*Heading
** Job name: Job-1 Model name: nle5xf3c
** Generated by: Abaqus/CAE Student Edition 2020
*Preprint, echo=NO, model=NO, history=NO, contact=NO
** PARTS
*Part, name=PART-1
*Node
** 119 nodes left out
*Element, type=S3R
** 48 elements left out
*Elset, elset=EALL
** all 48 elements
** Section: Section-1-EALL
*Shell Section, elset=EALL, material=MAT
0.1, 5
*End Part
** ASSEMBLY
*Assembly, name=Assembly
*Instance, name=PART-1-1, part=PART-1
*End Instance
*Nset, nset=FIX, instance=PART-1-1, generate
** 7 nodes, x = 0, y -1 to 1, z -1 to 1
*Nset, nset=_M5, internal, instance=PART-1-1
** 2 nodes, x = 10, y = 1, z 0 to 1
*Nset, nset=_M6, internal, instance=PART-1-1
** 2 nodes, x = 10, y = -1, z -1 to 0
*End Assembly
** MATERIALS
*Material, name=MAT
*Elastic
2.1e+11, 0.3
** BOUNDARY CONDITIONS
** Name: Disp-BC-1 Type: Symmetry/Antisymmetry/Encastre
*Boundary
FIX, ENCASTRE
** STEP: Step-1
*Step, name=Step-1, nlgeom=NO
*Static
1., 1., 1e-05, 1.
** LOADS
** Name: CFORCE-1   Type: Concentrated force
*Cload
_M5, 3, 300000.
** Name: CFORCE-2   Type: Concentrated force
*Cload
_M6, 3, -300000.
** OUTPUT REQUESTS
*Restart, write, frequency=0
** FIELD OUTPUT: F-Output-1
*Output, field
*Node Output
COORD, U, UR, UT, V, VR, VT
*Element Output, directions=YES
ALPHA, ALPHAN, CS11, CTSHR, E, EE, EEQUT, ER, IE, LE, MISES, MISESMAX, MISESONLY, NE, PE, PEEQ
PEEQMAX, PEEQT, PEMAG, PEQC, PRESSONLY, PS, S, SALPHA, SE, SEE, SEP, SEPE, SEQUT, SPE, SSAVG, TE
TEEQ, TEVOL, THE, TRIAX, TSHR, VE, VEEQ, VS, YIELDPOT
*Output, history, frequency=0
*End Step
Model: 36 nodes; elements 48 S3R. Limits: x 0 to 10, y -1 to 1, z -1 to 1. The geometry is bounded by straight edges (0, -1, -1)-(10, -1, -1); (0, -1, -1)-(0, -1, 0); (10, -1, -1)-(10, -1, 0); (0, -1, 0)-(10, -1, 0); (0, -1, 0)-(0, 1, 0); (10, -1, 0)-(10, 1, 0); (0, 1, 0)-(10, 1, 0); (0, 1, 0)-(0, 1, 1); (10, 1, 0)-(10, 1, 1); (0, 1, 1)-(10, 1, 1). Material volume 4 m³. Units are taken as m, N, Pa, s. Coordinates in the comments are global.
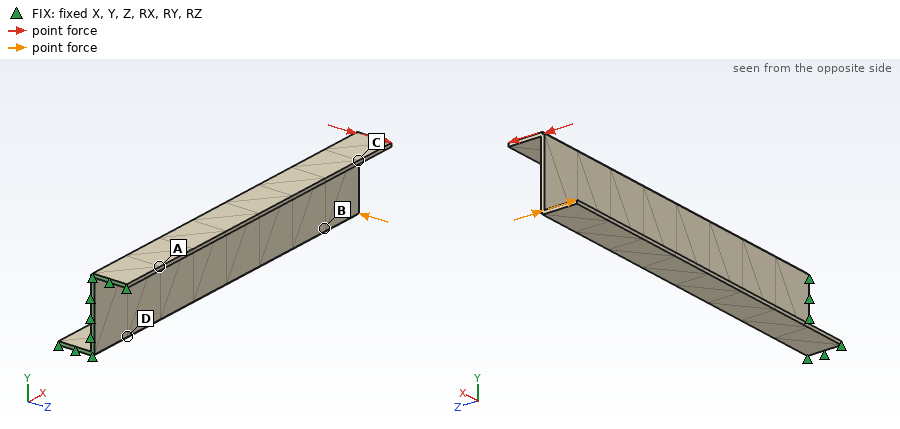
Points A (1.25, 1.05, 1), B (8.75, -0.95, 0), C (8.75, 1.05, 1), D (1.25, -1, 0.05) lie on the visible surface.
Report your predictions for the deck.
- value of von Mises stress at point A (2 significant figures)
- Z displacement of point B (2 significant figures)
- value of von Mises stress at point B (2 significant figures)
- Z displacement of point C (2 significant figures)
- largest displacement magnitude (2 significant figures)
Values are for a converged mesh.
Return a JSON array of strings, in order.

["1.3e+08 Pa", "-0.025 m", "4.3e+07 Pa", "0.027 m", "0.044 m"]
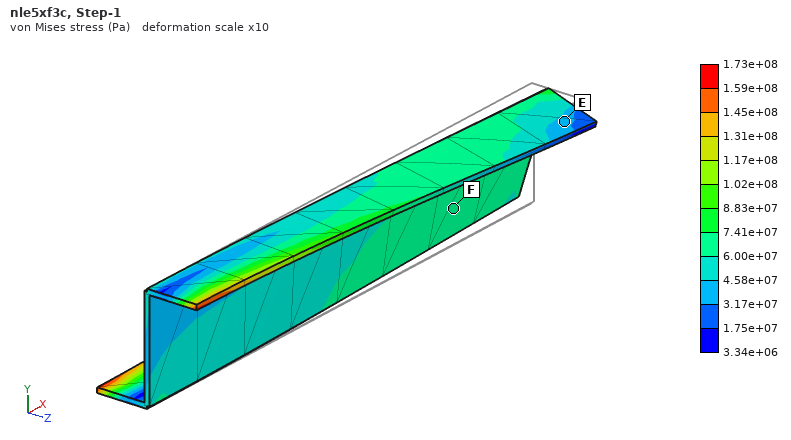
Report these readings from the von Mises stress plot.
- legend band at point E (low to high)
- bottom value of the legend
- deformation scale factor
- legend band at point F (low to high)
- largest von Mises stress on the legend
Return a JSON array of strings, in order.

["3.17e+07 to 4.58e+07 Pa", "3.34e+06 Pa", "10", "6.00e+07 to 7.41e+07 Pa", "1.73e+08 Pa"]
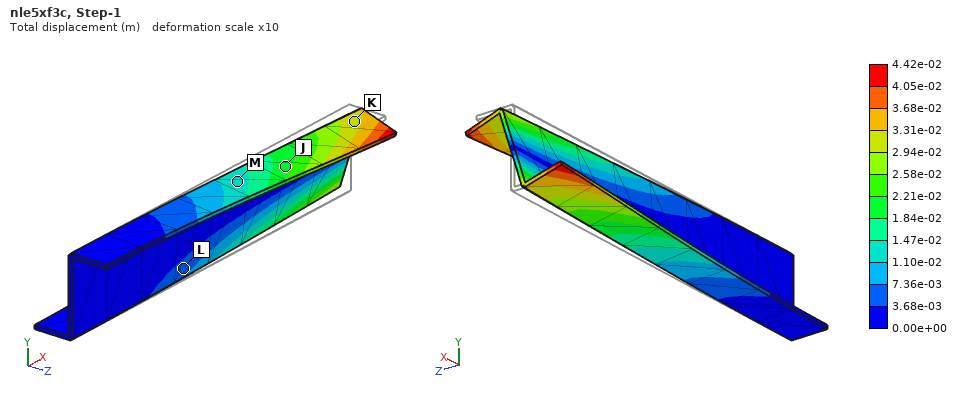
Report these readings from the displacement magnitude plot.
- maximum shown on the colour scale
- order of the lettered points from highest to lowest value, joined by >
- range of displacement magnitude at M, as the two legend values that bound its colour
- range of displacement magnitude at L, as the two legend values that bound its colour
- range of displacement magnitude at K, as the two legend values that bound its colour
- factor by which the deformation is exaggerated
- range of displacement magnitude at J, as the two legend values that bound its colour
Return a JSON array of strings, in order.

["4.42e-02 m", "K > J > M > L", "1.10e-02 to 1.47e-02 m", "3.68e-03 to 7.36e-03 m", "2.94e-02 to 3.31e-02 m", "10", "1.84e-02 to 2.21e-02 m"]
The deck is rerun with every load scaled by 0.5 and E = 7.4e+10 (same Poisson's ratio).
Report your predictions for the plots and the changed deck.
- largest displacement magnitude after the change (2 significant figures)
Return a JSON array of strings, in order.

["0.063 m"]
